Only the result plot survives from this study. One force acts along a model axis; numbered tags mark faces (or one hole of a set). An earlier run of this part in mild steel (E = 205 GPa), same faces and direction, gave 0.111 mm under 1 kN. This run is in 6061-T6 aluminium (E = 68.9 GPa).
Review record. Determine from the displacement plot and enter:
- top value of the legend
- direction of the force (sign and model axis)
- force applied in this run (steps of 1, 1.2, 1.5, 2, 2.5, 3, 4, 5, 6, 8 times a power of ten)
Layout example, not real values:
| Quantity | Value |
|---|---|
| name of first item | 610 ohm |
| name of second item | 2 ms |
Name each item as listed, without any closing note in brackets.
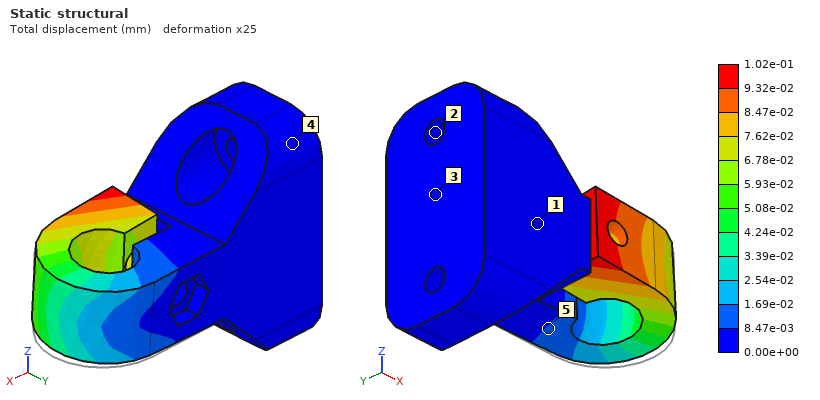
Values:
| Quantity | Value |
|---|---|
| top value of the legend | 1.02e-01 mm |
| direction of the force | +Z |
| force applied in this run | 300 N |
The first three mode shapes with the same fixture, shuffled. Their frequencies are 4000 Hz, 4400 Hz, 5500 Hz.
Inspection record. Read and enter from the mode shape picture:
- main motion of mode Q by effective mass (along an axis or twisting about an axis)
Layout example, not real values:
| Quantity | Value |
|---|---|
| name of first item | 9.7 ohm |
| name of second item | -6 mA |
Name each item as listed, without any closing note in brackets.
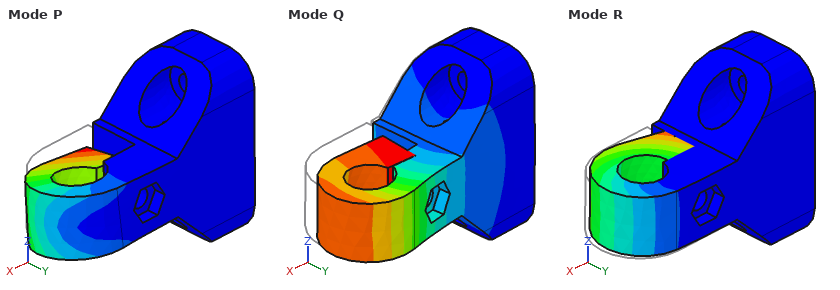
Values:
| Quantity | Value |
|---|---|
| main motion of mode Q by effective mass | along Y |
